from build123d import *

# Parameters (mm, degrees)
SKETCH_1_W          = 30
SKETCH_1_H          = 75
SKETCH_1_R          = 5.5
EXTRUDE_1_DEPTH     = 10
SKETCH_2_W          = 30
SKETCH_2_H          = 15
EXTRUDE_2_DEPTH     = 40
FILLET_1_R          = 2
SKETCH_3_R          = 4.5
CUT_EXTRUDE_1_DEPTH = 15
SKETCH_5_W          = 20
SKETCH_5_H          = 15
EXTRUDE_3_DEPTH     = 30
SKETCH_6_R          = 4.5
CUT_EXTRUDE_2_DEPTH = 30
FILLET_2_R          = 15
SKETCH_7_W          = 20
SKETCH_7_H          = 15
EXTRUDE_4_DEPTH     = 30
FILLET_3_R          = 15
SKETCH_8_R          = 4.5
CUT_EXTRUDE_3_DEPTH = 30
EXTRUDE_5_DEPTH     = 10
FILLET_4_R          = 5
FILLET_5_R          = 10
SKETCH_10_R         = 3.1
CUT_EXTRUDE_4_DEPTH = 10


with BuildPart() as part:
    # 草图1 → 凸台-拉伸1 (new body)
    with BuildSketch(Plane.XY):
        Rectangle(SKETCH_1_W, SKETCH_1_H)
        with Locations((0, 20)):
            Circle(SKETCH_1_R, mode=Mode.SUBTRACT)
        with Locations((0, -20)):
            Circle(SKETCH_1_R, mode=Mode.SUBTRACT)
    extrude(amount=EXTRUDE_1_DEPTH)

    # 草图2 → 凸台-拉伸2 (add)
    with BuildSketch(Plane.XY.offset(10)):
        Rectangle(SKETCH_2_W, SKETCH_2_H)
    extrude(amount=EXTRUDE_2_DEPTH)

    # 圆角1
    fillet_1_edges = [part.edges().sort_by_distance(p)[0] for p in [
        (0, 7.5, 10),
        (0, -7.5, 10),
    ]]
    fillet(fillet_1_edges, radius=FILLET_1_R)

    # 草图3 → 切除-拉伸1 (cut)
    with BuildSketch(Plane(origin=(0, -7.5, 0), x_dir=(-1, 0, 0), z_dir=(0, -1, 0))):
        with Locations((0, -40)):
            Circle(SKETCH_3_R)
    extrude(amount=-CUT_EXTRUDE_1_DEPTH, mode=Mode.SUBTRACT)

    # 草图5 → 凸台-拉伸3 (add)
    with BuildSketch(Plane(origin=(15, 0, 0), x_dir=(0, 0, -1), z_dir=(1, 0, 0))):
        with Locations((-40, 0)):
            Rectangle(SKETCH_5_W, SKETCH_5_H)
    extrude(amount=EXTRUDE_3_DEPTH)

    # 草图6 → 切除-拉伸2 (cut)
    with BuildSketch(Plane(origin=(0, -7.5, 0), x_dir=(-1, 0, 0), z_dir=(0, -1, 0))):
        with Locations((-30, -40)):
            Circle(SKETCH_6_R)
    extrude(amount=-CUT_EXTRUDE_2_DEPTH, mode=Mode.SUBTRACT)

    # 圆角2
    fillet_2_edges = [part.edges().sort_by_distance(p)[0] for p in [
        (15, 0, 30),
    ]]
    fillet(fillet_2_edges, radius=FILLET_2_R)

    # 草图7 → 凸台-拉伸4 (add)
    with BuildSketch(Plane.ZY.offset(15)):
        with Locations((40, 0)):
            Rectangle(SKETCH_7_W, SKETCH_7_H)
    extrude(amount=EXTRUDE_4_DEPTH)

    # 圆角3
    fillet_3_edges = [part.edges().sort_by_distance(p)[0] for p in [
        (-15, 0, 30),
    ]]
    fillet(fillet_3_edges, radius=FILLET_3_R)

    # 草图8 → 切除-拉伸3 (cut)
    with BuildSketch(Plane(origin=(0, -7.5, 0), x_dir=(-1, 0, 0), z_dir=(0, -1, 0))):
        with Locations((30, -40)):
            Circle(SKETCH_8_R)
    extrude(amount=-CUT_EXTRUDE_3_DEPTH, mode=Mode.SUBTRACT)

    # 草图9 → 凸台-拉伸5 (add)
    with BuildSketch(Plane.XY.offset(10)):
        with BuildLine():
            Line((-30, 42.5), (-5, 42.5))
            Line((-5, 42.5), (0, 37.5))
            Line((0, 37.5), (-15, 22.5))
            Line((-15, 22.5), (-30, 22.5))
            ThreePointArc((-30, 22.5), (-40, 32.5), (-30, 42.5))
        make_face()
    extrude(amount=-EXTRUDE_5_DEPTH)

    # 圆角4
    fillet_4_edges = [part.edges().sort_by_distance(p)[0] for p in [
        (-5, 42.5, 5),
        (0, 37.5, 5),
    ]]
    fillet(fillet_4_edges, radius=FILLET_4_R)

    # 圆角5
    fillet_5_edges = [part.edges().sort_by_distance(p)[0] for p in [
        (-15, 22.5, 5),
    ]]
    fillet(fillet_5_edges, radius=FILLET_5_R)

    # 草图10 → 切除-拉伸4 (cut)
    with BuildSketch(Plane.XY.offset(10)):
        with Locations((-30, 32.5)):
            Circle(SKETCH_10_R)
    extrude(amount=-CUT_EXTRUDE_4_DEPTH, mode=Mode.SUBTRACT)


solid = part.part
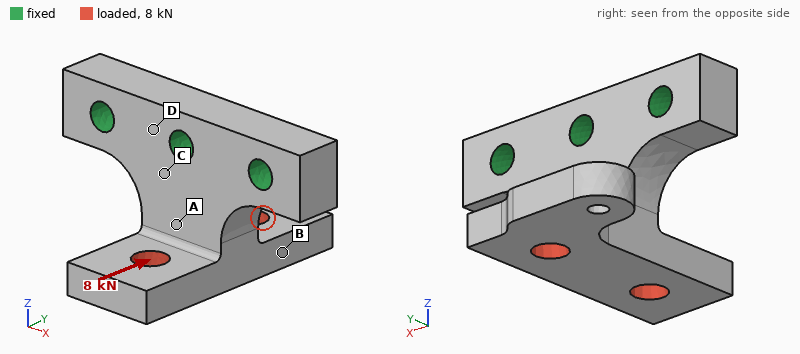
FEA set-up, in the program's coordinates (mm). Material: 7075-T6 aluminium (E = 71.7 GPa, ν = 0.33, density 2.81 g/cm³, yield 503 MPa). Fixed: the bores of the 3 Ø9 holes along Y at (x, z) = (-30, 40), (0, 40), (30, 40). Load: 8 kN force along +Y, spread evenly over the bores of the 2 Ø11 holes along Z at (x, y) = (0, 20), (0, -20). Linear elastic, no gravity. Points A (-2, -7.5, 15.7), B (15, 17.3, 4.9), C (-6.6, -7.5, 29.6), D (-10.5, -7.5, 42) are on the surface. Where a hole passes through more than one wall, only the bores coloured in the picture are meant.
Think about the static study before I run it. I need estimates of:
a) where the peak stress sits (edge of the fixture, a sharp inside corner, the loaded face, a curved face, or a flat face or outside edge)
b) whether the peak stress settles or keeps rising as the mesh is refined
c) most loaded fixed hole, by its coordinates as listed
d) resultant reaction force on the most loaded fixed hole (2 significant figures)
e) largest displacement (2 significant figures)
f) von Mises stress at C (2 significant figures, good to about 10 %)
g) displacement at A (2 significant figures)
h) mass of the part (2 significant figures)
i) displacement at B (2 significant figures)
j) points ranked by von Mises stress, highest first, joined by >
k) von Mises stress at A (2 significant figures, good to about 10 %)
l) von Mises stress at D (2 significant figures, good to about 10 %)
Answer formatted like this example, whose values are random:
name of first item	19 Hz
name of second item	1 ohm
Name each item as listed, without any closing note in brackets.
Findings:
where the peak stress sits	edge of the fixture
whether the peak stress settles or keeps rising as the mesh is refined	keeps rising
most loaded fixed hole, by its coordinates as listed	(0, 40)
resultant reaction force on the most loaded fixed hole	6.9 kN
largest displacement	0.33 mm
von Mises stress at C	120 MPa
displacement at A	0.095 mm
mass of the part	170 g
displacement at B	0.19 mm
points ranked by von Mises stress, highest first, joined by >	C > A > D > B
von Mises stress at A	68 MPa
von Mises stress at D	40 MPa
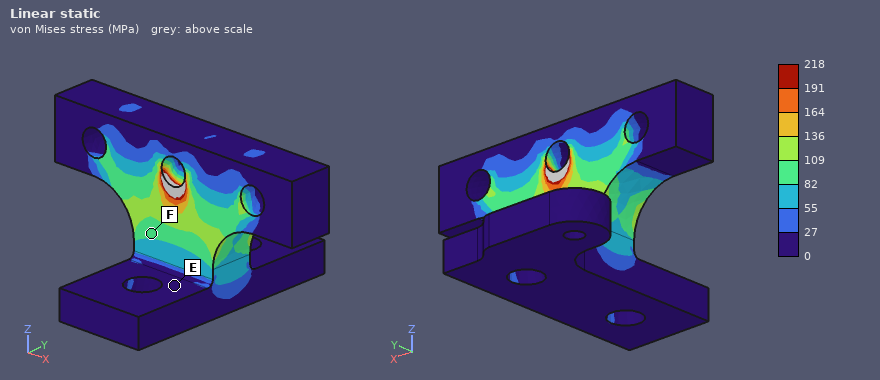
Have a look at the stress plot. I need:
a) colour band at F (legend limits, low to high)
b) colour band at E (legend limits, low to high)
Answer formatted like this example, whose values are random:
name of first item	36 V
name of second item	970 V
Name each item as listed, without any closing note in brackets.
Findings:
colour band at F	82 to 109 MPa
colour band at E	0 to 27 MPa
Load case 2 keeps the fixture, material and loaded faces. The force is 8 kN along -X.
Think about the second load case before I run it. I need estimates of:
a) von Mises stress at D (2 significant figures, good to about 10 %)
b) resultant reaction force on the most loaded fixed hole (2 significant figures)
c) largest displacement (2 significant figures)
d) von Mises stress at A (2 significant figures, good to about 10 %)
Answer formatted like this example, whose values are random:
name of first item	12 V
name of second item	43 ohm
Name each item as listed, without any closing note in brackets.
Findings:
von Mises stress at D	12 MPa
resultant reaction force on the most loaded fixed hole	5.6 kN
largest displacement	79 µm
von Mises stress at A	41 MPa
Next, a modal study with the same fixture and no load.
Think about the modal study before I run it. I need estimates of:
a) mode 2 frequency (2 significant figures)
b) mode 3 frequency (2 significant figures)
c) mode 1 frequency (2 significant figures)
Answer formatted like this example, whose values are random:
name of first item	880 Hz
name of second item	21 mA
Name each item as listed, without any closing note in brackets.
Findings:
mode 2 frequency	3400 Hz
mode 3 frequency	4300 Hz
mode 1 frequency	2400 Hz
